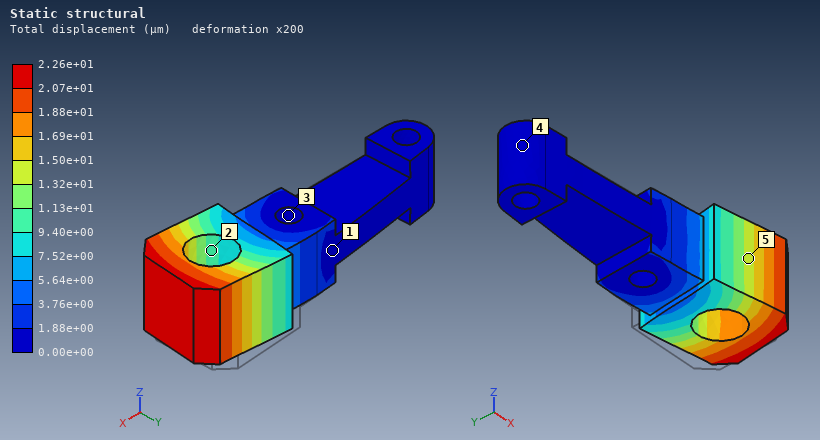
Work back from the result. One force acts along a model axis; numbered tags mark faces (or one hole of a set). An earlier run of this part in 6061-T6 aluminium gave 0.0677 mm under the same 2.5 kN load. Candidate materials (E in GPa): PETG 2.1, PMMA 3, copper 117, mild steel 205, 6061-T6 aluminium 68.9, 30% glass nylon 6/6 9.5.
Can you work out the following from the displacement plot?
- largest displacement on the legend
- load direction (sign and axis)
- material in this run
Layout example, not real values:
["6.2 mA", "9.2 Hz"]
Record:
["2.26e+01 µm", "-Y", "mild steel"]
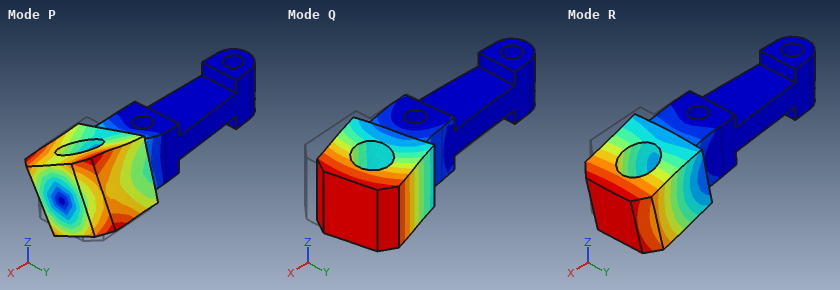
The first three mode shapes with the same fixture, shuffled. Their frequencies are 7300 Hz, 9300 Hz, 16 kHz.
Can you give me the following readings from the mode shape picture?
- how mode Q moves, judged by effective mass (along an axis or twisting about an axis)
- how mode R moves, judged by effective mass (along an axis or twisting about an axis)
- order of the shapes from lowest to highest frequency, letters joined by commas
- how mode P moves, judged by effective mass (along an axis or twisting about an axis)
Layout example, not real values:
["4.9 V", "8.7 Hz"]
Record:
["along Y", "along Z", "Q, R, P", "twisting about X"]
